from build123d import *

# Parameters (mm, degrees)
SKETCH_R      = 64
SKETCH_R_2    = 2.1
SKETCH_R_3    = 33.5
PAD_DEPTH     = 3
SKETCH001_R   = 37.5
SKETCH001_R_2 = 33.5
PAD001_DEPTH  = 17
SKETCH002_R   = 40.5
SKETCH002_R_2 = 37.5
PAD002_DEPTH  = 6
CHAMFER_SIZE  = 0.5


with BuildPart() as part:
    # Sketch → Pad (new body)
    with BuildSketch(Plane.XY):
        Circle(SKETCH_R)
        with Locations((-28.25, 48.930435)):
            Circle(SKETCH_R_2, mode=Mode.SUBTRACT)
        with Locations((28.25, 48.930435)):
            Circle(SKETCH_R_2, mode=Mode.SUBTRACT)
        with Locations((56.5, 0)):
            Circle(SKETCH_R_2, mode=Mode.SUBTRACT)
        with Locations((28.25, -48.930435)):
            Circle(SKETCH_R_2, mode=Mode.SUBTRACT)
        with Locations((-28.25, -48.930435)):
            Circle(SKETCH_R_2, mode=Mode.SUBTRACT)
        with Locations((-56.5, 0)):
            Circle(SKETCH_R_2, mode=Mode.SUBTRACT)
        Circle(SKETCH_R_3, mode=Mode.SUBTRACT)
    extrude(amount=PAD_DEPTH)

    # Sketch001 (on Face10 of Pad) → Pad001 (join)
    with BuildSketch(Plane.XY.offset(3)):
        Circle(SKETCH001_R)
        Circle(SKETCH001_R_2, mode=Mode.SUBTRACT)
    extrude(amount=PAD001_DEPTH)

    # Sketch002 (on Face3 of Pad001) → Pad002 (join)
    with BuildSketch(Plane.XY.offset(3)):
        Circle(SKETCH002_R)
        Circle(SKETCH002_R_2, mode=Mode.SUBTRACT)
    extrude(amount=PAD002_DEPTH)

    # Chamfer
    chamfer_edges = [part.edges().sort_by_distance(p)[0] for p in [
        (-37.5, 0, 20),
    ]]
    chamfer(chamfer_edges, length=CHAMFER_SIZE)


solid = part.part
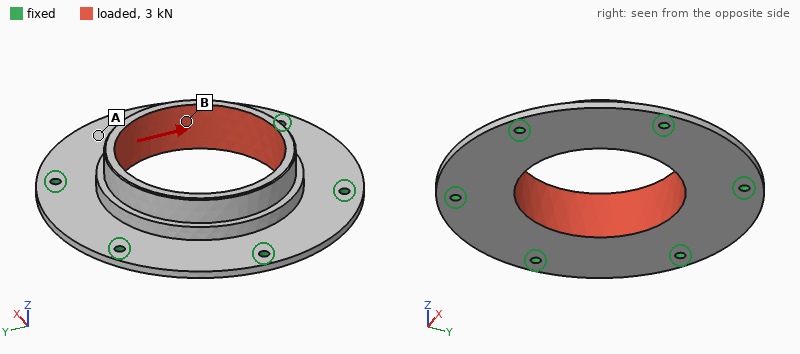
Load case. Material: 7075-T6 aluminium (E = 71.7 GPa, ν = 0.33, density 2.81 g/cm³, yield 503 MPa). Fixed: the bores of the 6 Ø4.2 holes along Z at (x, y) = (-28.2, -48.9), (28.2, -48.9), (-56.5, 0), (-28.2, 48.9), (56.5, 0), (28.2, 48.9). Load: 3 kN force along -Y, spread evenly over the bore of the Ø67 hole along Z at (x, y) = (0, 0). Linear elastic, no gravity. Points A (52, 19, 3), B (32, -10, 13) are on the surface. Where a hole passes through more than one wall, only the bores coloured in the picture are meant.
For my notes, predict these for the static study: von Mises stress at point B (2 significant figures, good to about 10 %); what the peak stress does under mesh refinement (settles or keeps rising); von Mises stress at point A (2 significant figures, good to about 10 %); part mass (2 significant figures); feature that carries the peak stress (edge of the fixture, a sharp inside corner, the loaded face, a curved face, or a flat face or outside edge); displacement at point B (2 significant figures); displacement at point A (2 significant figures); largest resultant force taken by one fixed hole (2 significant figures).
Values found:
4.8 MPa
keeps rising
2.6 MPa
130 g
edge of the fixture
8.3 µm
4.5 µm
560 N
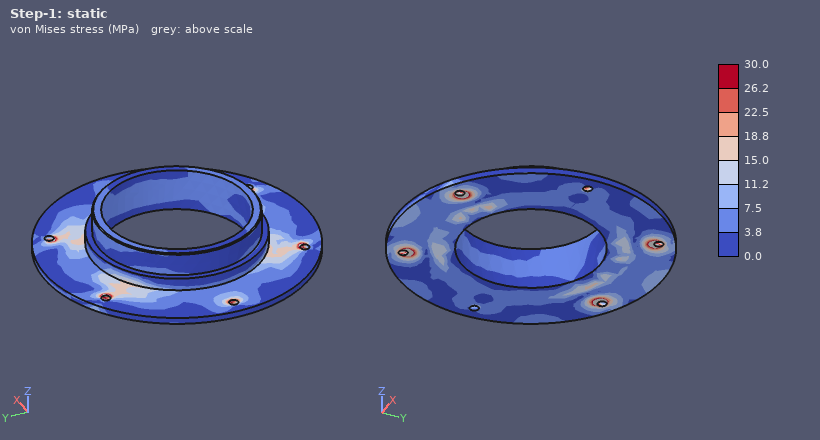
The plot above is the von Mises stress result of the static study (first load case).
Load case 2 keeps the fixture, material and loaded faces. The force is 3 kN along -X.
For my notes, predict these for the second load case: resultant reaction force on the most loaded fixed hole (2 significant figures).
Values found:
600 N
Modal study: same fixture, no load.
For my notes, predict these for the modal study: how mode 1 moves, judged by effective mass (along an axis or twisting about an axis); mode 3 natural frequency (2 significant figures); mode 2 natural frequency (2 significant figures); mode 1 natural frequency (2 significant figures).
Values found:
along Z
4500 Hz
4500 Hz
3700 Hz
